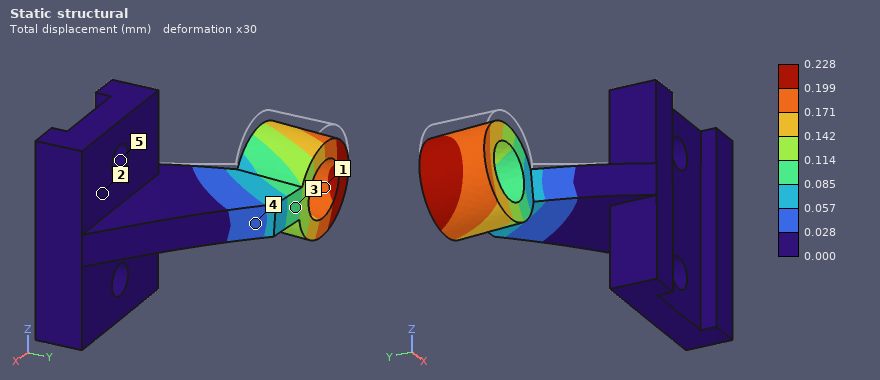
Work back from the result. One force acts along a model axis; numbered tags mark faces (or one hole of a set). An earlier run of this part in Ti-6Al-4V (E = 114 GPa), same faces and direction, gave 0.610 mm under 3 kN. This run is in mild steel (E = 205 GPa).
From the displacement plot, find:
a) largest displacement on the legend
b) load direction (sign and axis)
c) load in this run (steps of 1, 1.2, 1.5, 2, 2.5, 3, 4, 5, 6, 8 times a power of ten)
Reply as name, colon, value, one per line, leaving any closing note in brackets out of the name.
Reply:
largest displacement on the legend: 0.228 mm
load direction: -Z
load in this run: 2 kN
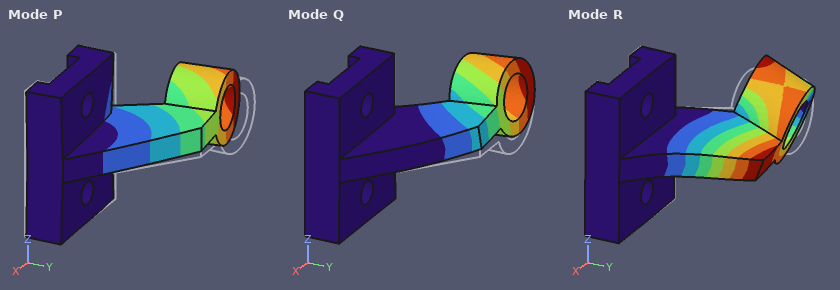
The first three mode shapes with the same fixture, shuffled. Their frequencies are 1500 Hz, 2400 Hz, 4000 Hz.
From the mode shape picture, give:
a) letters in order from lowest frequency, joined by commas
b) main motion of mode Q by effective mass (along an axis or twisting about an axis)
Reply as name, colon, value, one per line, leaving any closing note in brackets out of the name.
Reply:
letters in order from lowest frequency, joined by commas: Q, P, R
main motion of mode Q by effective mass: along Z
